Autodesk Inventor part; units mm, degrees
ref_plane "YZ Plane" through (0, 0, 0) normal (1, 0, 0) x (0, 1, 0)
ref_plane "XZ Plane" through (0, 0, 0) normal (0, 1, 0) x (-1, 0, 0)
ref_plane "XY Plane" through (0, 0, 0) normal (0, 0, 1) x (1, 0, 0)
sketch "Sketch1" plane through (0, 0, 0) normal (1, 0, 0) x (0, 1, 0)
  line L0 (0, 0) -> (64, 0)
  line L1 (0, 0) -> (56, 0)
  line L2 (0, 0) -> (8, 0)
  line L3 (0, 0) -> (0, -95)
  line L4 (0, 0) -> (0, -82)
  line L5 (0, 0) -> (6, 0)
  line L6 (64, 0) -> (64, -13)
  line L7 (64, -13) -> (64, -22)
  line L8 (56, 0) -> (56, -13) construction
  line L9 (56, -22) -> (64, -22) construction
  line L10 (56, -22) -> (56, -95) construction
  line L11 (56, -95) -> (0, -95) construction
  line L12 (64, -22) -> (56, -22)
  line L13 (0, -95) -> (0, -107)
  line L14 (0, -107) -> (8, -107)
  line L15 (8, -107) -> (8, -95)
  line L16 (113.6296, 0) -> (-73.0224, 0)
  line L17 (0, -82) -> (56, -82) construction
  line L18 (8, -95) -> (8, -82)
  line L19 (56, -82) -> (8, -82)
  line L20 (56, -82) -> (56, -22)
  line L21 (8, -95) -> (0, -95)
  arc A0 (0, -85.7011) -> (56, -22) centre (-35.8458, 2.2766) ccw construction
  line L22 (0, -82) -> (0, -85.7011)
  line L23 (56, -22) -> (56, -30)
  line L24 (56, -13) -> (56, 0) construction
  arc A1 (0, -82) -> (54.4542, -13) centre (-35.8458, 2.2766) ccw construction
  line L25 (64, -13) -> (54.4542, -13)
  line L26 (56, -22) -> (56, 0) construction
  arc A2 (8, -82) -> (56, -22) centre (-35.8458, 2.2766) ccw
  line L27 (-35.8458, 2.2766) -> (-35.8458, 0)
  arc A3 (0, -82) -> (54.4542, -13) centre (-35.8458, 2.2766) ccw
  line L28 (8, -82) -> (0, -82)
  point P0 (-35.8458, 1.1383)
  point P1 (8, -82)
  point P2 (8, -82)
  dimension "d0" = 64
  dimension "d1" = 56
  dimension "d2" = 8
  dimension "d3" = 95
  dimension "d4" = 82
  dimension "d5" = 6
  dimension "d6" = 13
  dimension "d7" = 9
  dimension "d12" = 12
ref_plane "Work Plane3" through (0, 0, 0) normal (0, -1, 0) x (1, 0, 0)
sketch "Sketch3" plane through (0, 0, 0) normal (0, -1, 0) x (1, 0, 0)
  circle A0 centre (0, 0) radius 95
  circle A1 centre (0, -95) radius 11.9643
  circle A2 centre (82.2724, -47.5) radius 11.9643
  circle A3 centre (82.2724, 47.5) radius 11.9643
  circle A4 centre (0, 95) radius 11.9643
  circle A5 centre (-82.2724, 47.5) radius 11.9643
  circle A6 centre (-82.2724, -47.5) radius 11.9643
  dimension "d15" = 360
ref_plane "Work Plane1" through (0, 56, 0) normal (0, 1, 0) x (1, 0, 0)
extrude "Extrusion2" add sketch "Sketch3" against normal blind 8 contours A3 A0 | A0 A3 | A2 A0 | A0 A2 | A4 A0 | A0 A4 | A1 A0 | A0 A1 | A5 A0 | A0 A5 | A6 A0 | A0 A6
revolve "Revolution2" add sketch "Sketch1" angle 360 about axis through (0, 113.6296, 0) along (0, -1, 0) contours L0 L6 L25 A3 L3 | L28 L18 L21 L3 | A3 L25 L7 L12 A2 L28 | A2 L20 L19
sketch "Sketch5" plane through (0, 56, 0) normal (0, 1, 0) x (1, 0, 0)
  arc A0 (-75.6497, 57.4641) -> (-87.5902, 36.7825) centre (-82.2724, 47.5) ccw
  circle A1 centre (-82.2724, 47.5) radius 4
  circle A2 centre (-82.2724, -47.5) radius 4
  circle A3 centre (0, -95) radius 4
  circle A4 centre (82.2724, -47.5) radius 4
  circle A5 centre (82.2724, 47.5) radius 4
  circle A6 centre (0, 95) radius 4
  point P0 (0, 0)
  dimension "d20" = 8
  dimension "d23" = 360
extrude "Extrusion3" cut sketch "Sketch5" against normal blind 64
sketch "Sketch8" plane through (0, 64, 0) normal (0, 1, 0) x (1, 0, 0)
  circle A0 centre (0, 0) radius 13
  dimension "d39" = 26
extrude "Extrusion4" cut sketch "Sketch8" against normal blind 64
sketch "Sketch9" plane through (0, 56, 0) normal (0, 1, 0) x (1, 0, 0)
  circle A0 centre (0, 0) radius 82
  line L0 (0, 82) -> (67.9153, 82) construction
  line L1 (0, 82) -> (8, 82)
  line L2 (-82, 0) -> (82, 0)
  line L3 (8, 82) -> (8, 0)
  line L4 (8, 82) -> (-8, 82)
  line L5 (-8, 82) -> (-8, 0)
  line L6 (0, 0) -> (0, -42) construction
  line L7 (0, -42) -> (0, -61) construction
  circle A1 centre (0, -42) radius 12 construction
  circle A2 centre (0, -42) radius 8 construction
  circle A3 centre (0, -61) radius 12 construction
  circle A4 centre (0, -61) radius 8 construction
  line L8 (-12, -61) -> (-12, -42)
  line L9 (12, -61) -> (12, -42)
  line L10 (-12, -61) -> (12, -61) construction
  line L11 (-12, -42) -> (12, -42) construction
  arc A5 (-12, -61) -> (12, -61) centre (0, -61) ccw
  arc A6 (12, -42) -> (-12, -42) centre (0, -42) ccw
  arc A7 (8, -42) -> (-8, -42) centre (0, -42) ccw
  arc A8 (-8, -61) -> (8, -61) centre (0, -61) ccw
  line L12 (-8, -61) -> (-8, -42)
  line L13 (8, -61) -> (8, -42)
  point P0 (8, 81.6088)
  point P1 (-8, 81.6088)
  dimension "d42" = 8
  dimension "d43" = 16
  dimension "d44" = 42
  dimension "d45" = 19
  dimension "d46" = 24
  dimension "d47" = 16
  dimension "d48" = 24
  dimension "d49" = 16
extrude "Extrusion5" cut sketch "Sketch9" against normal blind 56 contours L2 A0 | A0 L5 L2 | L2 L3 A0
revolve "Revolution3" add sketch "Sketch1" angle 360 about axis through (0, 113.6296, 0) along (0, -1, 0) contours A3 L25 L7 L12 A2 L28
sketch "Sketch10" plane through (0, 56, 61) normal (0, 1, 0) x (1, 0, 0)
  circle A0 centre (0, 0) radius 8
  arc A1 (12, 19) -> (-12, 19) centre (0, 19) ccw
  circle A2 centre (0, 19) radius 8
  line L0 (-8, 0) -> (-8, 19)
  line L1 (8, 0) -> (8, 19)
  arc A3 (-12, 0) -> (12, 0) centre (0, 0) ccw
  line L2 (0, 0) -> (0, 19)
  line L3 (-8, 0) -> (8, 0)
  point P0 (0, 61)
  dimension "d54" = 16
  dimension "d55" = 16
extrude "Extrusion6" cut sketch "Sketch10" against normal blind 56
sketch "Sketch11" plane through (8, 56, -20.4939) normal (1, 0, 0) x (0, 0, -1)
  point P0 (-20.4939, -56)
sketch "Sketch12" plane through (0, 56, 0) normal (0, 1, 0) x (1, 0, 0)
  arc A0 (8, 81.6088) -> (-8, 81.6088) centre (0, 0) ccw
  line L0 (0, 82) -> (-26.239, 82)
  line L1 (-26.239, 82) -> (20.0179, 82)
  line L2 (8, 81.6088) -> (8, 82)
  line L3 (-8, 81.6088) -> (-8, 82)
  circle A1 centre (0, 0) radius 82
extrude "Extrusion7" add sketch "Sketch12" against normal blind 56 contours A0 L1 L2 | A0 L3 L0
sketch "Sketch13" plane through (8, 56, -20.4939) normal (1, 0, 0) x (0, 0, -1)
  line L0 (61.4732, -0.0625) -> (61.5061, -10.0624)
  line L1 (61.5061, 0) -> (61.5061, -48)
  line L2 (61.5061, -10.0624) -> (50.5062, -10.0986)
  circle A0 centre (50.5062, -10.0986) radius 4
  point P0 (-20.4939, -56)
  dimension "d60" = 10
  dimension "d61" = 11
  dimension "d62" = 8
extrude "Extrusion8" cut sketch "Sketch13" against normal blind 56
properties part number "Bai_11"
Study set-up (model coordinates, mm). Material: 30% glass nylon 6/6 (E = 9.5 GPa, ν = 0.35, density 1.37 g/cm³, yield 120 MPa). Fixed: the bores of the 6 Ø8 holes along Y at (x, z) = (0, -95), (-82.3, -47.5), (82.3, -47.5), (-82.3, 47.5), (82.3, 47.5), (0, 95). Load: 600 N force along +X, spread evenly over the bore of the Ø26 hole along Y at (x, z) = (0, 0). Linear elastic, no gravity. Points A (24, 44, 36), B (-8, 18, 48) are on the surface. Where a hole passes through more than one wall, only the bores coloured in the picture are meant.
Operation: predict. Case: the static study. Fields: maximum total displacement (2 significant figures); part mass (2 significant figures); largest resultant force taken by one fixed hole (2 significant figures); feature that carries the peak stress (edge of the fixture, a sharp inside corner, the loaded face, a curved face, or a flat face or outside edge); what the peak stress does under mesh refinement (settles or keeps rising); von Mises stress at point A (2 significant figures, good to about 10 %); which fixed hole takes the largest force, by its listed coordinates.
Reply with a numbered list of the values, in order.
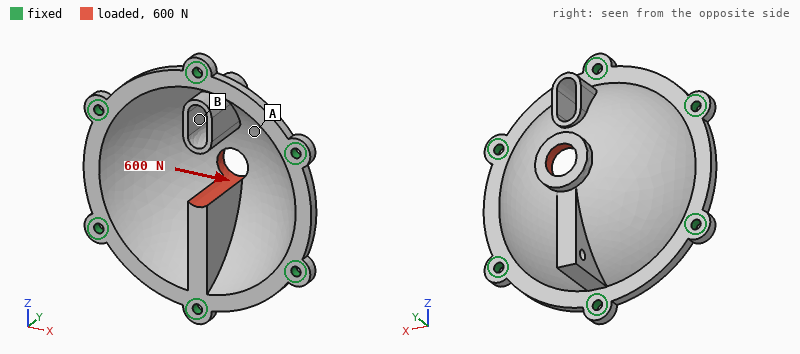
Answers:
1. 0.19 mm
2. 340 g
3. 240 N
4. a sharp inside corner
5. keeps rising
6. 1.2 MPa
7. (0, -95)
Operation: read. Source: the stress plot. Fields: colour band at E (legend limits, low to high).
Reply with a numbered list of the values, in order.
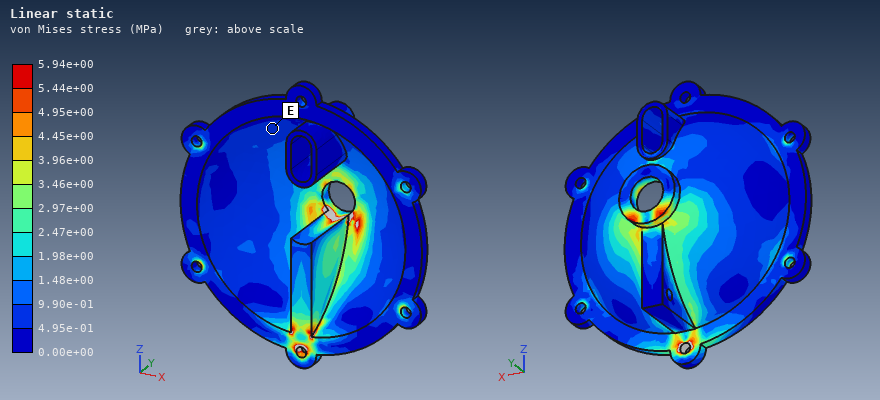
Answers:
1. 4.95e-01 to 9.90e-01 MPa
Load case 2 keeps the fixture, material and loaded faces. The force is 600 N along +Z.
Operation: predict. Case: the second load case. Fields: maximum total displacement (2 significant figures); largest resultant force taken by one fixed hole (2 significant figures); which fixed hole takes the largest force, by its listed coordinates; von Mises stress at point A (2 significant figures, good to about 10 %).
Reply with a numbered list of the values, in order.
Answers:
1. 17 µm
2. 310 N
3. (0, -95)
4. 0.72 MPa
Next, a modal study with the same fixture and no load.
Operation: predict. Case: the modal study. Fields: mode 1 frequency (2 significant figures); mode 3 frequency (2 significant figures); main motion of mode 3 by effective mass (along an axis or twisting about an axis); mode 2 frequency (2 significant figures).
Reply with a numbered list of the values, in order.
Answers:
1. 1500 Hz
2. 2100 Hz
3. along Y
4. 1900 Hz
